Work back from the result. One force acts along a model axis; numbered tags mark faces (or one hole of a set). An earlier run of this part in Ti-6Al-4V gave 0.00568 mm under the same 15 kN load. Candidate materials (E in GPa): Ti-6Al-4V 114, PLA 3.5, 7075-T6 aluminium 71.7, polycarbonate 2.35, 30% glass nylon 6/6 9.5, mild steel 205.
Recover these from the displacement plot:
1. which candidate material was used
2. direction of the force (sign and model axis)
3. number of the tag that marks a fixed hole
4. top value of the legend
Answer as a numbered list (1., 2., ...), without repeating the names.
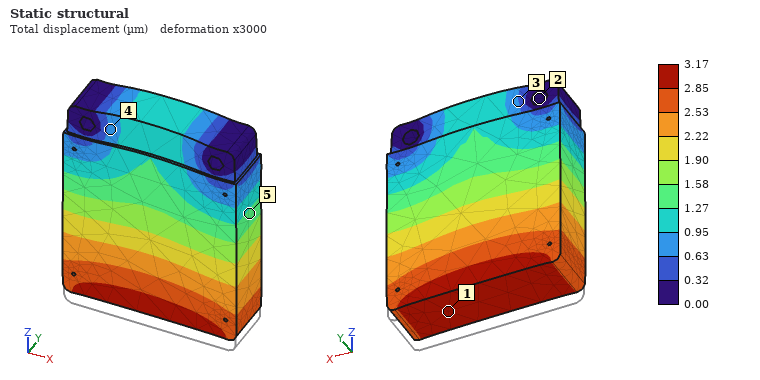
1. mild steel
2. +Z
3. 2
4. 3.17 µm
